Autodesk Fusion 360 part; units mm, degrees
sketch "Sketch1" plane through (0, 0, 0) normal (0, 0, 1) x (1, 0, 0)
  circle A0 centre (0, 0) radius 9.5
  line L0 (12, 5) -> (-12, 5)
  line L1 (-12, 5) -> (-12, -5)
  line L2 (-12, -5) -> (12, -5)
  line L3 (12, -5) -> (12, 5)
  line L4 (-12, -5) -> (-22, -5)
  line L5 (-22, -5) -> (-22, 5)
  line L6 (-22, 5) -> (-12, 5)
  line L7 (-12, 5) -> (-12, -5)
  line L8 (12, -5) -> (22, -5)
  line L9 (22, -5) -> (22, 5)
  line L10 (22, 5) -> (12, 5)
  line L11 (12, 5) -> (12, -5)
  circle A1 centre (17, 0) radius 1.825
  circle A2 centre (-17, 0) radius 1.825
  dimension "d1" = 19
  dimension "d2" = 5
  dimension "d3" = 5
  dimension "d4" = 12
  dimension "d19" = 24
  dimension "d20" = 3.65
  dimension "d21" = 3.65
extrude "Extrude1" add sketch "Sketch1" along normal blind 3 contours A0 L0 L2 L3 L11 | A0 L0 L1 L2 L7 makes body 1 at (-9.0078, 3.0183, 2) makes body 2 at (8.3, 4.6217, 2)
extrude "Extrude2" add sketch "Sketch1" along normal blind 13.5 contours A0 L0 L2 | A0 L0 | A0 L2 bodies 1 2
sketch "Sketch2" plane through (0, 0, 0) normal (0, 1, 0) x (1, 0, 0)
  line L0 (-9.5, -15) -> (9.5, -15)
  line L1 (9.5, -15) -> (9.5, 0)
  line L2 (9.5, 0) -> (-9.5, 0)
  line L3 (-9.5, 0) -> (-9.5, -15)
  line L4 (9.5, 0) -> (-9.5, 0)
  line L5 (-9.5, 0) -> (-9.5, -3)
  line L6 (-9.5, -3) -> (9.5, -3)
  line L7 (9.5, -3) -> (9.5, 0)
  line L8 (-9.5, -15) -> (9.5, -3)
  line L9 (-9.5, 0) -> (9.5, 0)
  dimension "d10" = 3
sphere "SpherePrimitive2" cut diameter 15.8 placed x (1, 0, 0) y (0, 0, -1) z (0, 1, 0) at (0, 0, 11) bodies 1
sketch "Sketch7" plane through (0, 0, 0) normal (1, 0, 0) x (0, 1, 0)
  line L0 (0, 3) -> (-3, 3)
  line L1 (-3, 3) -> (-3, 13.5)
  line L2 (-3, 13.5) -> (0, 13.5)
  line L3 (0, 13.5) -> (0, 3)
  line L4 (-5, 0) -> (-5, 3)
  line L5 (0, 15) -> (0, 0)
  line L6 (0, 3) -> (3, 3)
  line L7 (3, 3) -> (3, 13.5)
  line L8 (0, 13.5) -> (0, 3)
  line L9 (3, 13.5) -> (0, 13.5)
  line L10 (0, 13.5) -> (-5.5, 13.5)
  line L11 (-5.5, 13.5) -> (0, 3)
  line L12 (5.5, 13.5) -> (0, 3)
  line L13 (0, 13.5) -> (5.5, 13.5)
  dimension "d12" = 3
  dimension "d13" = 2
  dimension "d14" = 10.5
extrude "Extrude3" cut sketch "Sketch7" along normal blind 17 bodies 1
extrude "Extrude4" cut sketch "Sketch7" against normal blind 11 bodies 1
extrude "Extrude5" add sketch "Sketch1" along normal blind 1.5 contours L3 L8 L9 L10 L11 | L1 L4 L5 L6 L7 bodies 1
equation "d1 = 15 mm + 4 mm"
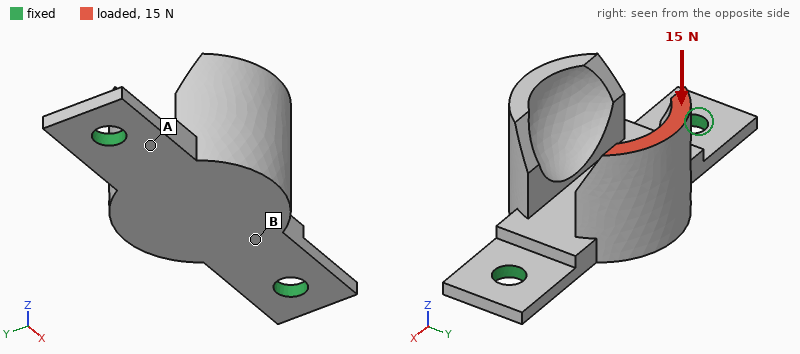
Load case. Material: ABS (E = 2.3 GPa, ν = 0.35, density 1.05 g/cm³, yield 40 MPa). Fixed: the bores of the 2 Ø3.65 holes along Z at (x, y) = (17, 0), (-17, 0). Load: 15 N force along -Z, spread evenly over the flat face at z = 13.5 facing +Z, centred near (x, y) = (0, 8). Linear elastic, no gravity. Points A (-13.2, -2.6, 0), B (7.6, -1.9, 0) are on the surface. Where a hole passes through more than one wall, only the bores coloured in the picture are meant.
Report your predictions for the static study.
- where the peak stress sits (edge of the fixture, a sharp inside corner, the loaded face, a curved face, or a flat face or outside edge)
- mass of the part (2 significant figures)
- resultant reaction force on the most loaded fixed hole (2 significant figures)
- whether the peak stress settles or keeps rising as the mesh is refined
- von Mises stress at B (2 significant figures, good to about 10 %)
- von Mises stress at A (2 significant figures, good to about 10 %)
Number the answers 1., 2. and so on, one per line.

1. edge of the fixture
2. 2.4 g
3. 13 N
4. keeps rising
5. 1.9 MPa
6. 5.5 MPa
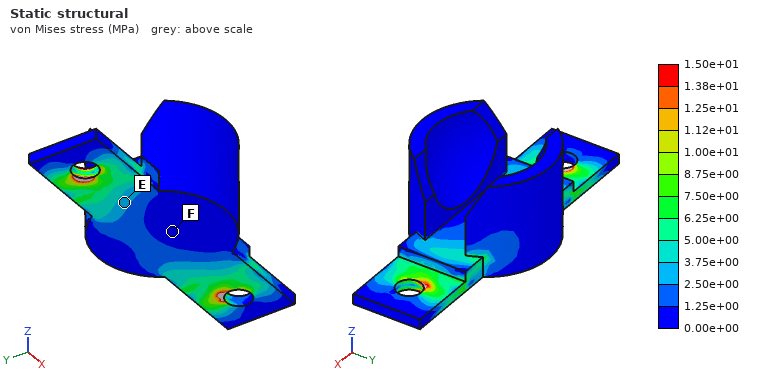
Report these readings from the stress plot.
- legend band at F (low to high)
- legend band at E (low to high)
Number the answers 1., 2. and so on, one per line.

1. 0.00e+00 to 1.25e+00 MPa
2. 2.50e+00 to 3.75e+00 MPa
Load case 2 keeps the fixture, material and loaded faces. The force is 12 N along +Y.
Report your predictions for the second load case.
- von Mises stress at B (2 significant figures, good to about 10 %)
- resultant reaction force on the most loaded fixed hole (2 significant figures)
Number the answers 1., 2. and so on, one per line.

1. 2.5 MPa
2. 6.6 N
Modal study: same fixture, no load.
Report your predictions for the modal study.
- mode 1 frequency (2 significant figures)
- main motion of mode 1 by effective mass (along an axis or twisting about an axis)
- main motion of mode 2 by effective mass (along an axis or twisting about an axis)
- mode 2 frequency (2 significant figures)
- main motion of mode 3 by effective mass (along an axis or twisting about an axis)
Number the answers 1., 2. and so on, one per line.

1. 1100 Hz
2. along Y
3. along Z
4. 2300 Hz
5. along X
